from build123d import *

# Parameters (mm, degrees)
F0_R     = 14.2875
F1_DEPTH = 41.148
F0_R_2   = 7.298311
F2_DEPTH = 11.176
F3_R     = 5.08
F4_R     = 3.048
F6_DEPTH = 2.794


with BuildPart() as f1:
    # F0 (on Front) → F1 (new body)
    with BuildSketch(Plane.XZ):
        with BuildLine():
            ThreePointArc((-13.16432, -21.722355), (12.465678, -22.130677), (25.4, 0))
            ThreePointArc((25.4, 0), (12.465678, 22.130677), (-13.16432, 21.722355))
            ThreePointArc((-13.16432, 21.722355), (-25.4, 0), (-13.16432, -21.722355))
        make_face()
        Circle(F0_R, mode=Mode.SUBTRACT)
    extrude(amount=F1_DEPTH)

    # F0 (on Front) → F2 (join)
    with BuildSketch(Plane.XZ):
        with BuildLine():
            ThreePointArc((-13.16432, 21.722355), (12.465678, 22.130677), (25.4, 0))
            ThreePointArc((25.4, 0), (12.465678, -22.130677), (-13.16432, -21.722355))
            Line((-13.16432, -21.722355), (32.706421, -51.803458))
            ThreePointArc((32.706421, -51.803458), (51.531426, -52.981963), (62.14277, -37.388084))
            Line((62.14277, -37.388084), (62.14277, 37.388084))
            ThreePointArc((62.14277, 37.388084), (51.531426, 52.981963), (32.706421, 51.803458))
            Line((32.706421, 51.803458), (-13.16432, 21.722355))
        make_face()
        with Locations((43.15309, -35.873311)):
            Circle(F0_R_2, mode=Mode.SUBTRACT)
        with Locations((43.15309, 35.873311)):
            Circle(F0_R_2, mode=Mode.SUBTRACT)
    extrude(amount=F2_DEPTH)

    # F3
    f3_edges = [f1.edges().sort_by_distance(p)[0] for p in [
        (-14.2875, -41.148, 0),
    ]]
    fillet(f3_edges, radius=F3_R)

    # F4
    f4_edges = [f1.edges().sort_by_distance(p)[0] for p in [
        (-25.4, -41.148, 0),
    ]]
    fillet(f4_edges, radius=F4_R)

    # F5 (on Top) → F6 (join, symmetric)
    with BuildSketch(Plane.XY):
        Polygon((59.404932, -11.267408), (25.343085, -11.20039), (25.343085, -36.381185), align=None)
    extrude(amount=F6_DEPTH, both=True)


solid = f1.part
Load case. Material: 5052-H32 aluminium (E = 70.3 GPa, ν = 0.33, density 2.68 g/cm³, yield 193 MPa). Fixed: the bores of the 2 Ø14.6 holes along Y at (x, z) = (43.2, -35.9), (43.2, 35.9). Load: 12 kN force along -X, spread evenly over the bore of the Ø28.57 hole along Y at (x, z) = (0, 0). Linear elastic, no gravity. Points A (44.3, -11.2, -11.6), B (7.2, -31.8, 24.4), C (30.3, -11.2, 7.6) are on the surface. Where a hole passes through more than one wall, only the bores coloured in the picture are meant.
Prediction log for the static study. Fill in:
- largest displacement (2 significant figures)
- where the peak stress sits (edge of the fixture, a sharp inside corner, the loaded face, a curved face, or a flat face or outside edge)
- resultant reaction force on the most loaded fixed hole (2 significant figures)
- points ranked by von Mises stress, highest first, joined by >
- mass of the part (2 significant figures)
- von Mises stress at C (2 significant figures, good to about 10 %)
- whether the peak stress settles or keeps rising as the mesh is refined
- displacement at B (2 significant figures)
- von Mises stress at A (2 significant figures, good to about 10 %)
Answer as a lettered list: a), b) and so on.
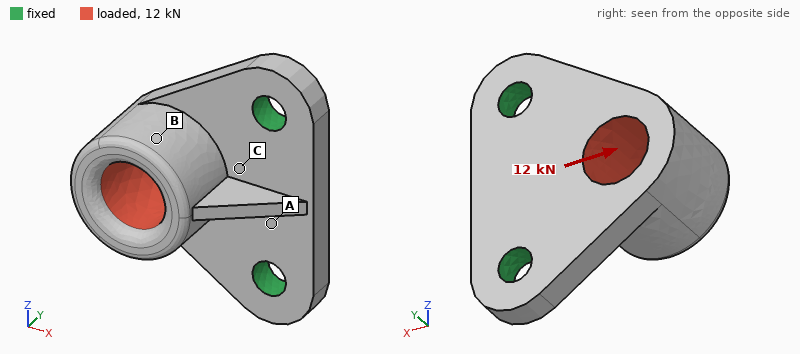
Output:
a) 0.37 mm
b) a sharp inside corner
c) 6.4 kN
d) C > A > B
e) 290 g
f) 73 MPa
g) keeps rising
h) 0.20 mm
i) 34 MPa
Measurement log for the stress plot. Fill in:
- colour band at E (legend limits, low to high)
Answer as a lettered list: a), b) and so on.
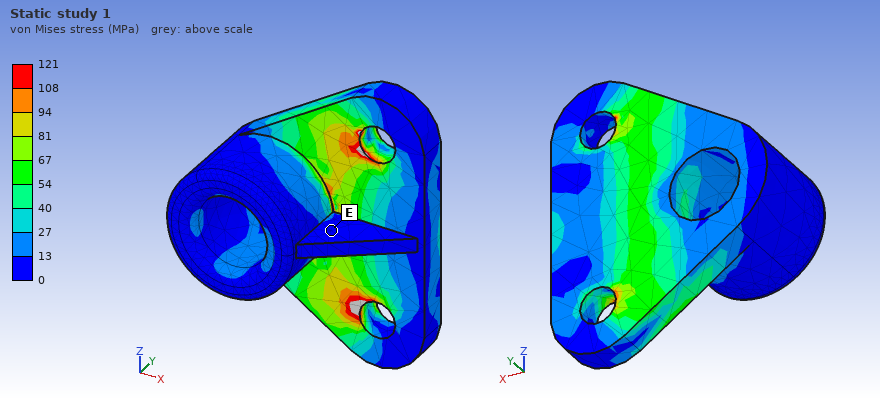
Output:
a) 0 to 13 MPa
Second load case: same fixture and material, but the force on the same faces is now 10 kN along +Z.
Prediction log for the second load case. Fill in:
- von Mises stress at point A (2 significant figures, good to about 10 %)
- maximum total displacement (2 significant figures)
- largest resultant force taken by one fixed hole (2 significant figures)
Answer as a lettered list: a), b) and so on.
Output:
a) 13 MPa
b) 71 µm
c) 7.5 kN
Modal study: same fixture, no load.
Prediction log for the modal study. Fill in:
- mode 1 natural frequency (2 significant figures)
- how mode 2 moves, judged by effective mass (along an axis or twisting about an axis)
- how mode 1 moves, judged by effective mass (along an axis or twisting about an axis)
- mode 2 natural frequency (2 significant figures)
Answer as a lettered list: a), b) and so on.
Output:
a) 1700 Hz
b) along Z
c) along Y
d) 4700 Hz
